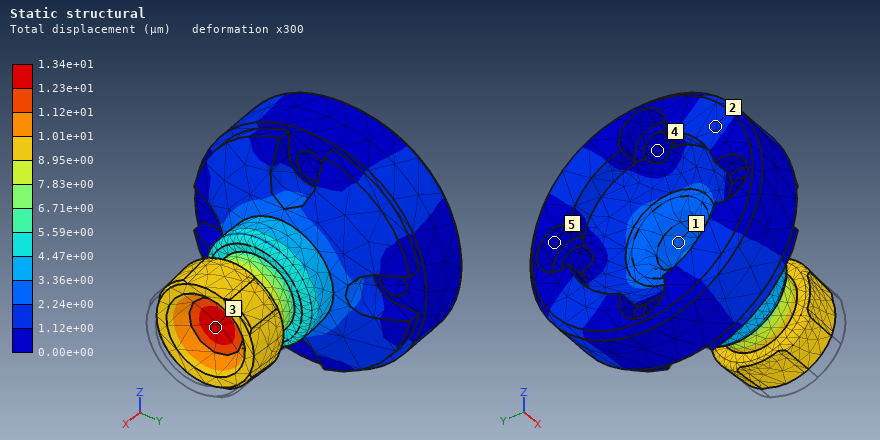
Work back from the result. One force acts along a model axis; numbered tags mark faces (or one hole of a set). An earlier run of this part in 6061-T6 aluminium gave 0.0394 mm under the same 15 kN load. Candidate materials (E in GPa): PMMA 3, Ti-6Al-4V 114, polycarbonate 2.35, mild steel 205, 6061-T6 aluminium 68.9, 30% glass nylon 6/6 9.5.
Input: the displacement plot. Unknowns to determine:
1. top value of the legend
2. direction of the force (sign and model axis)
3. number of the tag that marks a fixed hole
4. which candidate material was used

1.34e+01 µm
-X
4
mild steel
